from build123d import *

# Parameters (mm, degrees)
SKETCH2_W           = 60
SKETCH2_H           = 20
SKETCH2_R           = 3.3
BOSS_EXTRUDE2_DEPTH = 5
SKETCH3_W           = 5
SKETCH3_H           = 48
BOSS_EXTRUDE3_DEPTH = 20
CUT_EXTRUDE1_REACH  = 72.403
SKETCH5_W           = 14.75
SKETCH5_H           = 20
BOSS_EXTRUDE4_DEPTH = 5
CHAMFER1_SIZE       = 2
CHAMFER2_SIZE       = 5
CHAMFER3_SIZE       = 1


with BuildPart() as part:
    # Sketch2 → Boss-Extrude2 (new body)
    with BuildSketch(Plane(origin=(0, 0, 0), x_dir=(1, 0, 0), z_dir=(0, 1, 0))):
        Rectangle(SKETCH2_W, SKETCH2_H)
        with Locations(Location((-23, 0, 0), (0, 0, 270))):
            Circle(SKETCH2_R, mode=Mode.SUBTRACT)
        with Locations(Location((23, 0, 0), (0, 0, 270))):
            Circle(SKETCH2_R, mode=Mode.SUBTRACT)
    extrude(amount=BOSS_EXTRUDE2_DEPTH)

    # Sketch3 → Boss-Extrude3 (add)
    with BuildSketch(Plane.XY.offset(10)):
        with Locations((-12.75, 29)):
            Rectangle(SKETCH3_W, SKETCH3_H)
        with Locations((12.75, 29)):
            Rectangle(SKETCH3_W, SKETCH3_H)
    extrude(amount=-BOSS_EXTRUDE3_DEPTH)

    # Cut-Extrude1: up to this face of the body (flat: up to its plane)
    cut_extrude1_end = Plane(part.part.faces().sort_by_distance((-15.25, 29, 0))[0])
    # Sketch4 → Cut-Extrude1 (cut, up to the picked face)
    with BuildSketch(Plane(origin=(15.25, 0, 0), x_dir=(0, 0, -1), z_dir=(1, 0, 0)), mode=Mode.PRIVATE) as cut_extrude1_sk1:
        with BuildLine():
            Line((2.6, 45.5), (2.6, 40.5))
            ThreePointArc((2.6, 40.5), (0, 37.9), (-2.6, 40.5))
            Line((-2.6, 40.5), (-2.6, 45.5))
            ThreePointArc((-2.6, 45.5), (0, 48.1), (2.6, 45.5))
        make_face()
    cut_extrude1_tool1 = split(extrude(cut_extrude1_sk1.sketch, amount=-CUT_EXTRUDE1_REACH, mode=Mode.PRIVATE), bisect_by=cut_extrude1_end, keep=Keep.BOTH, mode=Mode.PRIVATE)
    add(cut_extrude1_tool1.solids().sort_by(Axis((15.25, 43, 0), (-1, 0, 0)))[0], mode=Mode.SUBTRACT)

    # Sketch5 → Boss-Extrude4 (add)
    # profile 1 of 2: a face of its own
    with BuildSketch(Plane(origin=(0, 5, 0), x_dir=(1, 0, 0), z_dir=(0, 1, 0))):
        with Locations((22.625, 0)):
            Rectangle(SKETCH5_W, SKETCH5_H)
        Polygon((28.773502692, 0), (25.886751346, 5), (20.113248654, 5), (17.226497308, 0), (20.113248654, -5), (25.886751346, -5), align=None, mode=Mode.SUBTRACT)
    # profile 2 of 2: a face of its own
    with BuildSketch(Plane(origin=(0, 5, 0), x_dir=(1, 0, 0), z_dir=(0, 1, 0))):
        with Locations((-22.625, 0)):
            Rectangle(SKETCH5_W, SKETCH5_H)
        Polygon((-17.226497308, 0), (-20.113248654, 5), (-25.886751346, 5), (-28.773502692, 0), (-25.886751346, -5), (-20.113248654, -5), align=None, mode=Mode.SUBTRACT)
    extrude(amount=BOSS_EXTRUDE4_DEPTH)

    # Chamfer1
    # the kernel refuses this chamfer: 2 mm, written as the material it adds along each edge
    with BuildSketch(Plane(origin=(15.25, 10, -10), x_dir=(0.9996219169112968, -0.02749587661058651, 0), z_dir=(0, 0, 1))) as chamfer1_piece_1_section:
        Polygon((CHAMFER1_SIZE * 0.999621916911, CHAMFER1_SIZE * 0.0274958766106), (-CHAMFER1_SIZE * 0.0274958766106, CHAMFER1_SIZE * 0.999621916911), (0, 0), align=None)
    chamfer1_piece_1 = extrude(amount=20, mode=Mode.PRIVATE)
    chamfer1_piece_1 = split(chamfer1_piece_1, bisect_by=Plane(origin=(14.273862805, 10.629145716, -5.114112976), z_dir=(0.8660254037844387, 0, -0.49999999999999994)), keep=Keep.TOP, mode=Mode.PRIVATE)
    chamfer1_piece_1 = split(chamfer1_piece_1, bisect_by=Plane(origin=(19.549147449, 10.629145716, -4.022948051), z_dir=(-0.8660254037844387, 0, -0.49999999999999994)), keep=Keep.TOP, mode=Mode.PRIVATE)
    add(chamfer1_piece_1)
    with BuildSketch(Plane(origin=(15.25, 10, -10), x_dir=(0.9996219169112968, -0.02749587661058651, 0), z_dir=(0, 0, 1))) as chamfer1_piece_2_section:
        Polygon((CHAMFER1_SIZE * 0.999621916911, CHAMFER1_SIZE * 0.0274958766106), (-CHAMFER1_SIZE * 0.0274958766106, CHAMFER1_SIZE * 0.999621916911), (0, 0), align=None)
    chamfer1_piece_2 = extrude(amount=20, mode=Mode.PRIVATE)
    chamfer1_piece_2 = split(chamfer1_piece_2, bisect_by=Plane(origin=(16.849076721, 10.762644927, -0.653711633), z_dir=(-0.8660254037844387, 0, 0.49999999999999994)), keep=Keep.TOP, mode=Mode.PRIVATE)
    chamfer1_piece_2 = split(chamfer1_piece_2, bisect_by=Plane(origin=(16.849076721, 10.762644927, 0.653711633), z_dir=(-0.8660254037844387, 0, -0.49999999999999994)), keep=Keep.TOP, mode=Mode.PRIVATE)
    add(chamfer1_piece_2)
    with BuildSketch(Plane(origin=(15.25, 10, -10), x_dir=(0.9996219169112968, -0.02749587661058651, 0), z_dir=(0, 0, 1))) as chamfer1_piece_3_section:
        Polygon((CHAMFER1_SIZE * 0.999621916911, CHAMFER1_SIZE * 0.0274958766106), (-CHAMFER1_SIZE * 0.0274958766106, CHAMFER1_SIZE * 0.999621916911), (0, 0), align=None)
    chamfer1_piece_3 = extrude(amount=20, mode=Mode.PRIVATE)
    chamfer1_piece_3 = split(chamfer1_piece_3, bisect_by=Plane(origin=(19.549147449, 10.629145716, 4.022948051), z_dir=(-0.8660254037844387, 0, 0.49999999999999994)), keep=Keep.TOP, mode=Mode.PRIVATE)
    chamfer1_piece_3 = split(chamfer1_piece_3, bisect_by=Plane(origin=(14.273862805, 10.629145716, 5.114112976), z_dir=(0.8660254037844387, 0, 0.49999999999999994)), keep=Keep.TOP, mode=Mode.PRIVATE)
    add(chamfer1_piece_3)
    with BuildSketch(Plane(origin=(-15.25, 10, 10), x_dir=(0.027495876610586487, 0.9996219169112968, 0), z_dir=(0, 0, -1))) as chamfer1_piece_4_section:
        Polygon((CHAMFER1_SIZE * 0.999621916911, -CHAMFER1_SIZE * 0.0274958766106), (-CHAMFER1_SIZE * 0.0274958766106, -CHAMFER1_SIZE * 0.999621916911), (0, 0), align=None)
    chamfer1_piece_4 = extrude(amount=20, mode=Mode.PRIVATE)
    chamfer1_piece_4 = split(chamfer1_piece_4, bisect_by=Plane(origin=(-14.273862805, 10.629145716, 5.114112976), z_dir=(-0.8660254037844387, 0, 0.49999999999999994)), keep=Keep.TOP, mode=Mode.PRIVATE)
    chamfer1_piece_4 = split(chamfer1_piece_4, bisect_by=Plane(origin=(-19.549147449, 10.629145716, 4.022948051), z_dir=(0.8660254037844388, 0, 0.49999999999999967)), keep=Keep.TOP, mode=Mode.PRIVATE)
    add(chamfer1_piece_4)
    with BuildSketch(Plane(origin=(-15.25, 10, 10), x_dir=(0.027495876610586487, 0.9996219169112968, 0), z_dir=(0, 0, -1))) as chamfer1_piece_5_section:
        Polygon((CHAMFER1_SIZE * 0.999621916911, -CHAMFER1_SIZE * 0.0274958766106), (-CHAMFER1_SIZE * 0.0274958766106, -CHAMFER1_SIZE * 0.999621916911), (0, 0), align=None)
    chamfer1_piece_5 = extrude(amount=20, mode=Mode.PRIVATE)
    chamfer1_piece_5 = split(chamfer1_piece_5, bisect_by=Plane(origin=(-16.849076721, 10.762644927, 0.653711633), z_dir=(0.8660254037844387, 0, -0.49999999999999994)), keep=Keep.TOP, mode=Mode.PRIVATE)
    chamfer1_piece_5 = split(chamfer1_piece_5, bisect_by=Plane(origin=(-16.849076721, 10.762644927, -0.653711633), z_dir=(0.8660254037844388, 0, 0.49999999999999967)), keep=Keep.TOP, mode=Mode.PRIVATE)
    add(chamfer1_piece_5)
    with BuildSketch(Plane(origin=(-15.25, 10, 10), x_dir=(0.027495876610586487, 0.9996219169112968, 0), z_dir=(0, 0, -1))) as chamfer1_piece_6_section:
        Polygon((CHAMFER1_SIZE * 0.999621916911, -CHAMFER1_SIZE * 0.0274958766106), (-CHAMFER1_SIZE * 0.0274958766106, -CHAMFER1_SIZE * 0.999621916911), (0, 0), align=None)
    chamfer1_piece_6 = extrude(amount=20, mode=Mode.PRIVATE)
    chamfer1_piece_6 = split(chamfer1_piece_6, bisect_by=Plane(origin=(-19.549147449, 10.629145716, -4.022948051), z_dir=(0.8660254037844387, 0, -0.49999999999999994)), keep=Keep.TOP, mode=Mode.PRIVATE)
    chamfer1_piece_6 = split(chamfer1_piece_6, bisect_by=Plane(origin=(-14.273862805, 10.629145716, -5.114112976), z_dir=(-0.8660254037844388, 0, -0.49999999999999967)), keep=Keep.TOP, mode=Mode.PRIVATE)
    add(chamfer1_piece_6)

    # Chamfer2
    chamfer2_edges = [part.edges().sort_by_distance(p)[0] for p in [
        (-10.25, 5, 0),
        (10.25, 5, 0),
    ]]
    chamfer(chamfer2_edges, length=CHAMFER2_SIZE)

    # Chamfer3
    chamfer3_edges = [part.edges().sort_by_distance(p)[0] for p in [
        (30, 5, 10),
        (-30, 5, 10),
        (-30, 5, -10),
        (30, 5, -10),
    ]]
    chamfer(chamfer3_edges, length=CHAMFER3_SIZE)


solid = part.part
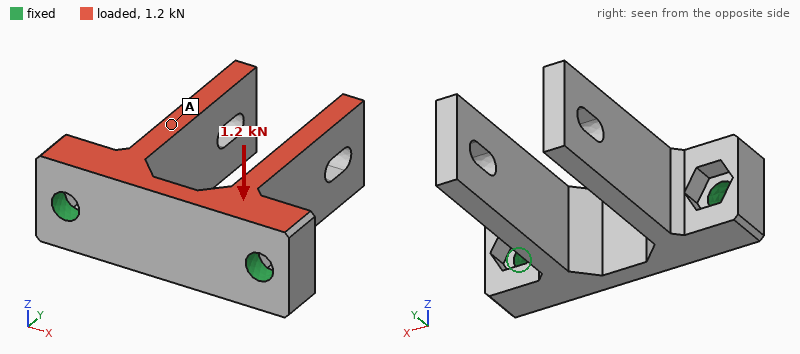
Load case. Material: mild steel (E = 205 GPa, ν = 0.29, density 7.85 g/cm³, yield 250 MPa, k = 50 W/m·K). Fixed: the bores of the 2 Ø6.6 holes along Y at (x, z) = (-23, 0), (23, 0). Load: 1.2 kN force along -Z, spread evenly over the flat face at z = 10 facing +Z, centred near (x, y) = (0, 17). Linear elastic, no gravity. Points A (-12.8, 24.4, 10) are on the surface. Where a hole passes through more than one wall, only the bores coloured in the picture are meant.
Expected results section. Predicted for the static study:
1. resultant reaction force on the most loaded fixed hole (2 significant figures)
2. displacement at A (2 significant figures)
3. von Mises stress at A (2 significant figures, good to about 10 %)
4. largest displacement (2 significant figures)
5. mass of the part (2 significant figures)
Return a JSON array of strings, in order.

["600 N", "11 µm", "8.5 MPa", "26 µm", "140 g"]
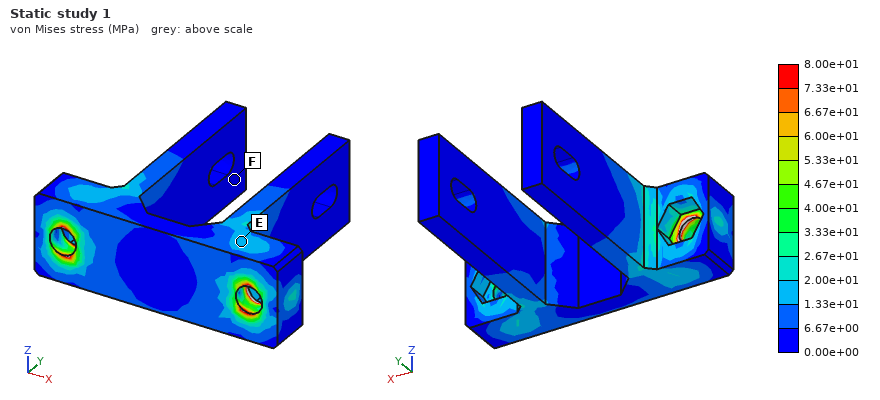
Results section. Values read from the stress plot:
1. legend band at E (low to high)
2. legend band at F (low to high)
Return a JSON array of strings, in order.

["1.33e+01 to 2.00e+01 MPa", "0.00e+00 to 6.67e+00 MPa"]
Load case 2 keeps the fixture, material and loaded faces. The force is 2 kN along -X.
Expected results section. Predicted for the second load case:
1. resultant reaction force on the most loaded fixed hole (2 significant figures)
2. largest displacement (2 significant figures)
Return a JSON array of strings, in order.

["1.2 kN", "0.14 mm"]
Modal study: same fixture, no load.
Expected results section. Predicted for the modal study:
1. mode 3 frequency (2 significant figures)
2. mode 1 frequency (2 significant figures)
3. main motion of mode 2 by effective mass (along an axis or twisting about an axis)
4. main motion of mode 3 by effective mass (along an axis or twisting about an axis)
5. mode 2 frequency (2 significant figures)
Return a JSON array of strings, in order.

["3700 Hz", "2000 Hz", "along X", "along Z", "2200 Hz"]
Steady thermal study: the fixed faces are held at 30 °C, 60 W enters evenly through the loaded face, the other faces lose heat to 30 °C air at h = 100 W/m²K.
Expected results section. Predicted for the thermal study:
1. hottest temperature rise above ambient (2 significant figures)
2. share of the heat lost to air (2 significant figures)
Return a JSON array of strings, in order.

["55 K", "33 %"]
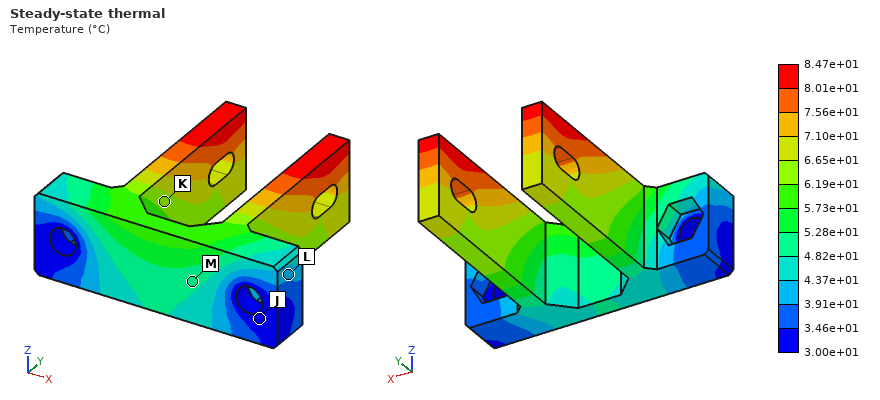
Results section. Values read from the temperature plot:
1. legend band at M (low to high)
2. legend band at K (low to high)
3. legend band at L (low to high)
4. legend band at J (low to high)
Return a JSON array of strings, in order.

["4.82e+01 to 5.28e+01 °C", "6.19e+01 to 6.65e+01 °C", "3.91e+01 to 4.37e+01 °C", "3.00e+01 to 3.46e+01 °C"]
